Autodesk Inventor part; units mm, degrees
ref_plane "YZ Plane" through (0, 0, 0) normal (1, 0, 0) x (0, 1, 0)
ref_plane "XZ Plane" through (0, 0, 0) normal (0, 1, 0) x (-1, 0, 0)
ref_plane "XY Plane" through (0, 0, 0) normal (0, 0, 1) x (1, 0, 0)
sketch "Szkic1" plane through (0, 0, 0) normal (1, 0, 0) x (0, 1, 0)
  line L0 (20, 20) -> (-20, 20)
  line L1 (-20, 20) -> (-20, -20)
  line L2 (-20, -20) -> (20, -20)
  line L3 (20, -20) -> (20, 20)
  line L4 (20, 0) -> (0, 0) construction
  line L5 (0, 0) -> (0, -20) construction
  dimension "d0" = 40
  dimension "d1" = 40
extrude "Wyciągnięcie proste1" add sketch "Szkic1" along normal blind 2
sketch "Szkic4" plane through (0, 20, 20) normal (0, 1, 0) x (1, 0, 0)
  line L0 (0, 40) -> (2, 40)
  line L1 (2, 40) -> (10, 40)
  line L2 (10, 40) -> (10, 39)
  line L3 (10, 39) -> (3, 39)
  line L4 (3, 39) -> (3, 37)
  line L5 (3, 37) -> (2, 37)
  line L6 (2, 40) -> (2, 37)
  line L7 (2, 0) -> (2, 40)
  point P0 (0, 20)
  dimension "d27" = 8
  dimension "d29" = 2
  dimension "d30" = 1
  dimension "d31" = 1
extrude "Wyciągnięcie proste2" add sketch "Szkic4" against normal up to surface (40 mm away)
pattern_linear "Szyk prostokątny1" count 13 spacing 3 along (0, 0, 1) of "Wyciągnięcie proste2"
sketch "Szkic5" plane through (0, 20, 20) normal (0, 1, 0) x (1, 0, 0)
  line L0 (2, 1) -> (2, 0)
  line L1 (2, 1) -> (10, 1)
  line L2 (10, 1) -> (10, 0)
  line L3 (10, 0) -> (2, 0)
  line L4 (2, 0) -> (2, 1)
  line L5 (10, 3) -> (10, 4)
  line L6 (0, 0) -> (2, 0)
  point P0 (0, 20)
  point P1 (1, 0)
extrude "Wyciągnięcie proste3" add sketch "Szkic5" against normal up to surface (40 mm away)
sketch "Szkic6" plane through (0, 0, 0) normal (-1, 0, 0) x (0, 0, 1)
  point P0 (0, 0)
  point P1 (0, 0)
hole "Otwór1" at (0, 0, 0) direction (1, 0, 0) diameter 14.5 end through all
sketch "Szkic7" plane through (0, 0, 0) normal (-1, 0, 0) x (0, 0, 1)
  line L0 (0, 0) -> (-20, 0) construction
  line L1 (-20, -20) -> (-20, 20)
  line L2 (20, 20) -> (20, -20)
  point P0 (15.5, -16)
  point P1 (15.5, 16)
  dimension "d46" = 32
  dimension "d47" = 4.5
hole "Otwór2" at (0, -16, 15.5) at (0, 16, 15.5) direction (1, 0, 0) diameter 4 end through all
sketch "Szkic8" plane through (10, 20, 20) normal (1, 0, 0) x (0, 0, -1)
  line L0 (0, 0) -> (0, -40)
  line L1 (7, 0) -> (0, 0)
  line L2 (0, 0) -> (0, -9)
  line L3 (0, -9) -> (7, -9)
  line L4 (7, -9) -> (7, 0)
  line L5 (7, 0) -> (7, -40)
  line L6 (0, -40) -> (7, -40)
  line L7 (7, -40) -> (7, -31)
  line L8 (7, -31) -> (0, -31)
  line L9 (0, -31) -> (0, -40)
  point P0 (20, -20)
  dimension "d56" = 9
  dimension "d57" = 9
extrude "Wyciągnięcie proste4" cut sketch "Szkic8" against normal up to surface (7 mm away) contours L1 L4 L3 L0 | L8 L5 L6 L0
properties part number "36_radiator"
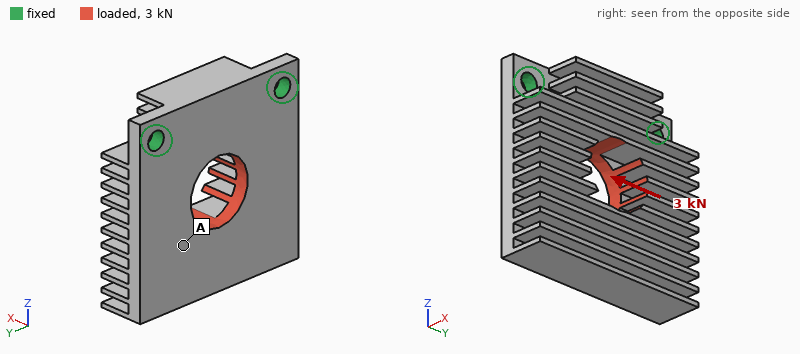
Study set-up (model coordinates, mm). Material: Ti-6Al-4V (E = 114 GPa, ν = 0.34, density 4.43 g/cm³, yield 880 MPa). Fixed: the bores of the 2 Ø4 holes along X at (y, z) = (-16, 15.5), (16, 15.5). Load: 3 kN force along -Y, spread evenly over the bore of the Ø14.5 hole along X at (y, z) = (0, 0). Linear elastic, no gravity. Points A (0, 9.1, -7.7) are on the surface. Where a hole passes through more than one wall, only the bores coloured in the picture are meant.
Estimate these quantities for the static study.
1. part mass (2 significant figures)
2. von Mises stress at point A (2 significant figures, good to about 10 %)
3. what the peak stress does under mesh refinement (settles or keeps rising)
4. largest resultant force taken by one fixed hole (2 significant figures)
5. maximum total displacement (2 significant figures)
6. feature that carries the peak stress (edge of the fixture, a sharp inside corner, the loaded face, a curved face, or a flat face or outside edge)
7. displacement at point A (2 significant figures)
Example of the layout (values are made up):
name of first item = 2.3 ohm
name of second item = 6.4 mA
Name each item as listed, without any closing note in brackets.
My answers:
part mass = 33 g
von Mises stress at point A = 22 MPa
what the peak stress does under mesh refinement = keeps rising
largest resultant force taken by one fixed hole = 2.0 kN
maximum total displacement = 94 µm
feature that carries the peak stress = edge of the fixture
displacement at point A = 32 µm
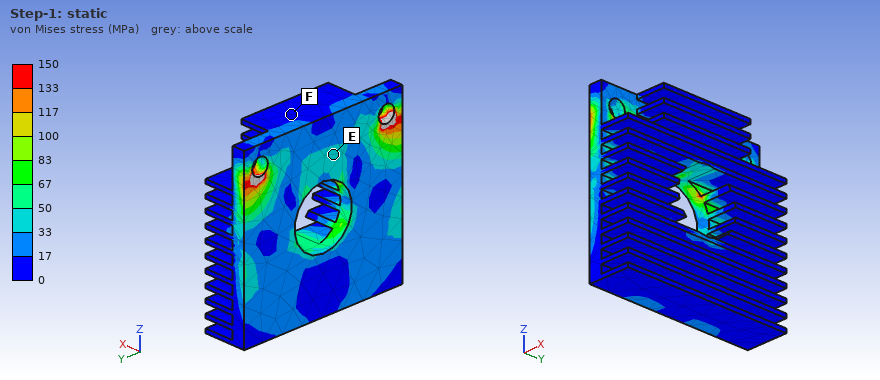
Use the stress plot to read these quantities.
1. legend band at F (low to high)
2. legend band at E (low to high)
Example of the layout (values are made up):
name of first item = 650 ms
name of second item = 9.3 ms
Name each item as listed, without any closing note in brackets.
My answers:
legend band at F = 0 to 17 MPa
legend band at E = 33 to 50 MPa
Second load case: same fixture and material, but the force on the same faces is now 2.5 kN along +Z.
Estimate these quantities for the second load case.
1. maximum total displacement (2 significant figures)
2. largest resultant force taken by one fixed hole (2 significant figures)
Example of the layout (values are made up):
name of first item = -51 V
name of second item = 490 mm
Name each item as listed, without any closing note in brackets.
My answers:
maximum total displacement = 0.28 mm
largest resultant force taken by one fixed hole = 1.3 kN
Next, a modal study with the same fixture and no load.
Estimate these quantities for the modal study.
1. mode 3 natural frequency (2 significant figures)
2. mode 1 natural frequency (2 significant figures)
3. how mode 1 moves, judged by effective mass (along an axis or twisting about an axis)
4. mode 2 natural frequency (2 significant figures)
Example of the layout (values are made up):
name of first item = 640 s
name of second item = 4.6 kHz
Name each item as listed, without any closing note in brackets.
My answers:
mode 3 natural frequency = 7300 Hz
mode 1 natural frequency = 1300 Hz
how mode 1 moves, judged by effective mass = along X
mode 2 natural frequency = 3100 Hz
